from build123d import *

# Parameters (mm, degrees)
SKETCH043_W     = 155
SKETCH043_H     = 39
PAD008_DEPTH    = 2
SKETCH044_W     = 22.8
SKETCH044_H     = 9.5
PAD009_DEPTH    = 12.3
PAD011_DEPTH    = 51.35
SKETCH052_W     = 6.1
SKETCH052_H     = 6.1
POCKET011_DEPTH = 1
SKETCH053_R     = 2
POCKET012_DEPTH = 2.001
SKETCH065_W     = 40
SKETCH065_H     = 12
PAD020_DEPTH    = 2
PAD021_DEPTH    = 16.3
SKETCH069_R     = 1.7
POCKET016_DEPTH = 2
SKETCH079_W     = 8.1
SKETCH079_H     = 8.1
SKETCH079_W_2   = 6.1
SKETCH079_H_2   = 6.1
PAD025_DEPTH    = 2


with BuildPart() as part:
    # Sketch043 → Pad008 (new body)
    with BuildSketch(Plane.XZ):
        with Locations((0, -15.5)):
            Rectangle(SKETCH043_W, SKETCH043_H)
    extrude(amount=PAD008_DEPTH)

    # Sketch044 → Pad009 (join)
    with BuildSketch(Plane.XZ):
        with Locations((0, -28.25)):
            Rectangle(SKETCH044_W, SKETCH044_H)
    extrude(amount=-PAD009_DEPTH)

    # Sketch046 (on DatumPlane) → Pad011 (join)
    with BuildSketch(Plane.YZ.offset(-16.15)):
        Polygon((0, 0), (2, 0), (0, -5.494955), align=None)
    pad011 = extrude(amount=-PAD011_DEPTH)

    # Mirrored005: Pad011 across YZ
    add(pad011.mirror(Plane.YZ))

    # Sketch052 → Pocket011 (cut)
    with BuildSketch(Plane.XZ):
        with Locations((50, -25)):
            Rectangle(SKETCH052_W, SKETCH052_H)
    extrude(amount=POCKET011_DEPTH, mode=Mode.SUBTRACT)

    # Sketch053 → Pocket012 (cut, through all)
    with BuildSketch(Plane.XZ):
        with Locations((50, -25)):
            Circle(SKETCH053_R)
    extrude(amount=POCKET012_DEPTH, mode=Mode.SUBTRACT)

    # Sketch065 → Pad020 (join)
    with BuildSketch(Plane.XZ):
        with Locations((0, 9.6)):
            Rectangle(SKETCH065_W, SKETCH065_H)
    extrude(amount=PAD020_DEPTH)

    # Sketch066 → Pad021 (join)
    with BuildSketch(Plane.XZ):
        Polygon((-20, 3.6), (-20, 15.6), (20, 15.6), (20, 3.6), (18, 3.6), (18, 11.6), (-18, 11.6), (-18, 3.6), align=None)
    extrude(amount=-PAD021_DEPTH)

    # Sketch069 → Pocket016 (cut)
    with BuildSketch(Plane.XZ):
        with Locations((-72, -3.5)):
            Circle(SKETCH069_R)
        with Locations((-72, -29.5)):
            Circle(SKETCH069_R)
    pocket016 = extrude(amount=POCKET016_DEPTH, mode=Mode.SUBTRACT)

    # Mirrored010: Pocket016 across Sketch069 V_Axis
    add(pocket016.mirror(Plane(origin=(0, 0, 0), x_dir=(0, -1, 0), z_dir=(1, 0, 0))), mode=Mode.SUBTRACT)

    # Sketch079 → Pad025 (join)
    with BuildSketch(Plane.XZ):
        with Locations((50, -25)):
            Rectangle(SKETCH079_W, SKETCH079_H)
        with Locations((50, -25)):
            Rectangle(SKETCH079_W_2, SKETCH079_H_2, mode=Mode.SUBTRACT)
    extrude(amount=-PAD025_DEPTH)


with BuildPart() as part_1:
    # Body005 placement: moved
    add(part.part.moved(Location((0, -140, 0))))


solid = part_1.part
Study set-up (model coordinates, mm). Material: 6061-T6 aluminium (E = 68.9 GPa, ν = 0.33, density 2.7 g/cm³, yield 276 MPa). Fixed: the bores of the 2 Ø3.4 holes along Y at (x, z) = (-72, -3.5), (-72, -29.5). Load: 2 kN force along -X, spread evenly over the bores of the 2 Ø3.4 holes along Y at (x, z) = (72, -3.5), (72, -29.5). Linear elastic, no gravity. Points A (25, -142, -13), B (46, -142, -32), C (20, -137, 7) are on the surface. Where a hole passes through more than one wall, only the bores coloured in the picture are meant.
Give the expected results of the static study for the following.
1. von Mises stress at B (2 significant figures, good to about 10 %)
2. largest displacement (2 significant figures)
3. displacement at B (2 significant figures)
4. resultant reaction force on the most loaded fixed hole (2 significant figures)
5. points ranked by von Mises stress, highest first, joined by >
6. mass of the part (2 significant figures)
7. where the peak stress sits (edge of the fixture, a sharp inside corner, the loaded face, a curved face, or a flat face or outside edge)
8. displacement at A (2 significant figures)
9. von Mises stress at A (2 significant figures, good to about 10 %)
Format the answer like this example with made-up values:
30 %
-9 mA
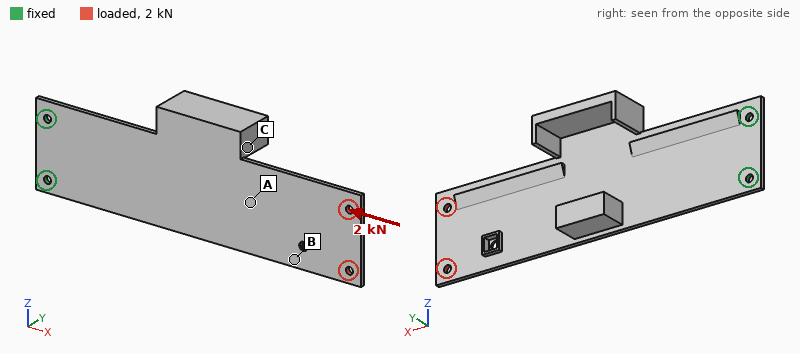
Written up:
39 MPa
0.55 mm
0.34 mm
1.0 kN
B > A > C
52 g
the loaded face
0.23 mm
26 MPa
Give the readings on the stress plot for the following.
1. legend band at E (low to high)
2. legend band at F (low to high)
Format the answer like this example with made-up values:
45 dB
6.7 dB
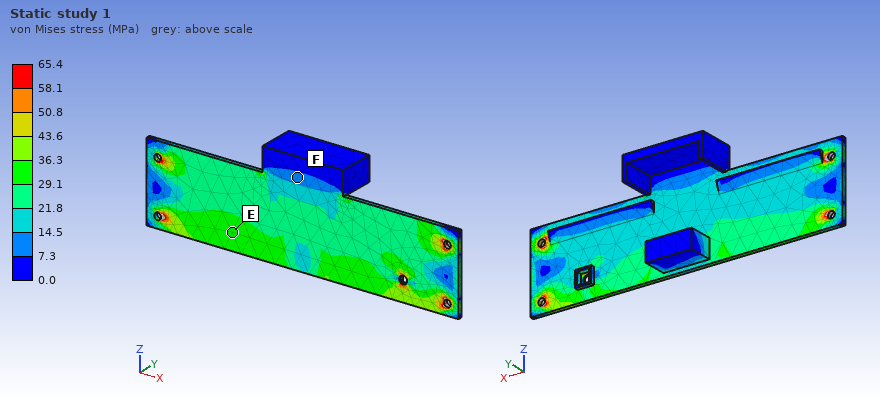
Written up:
29.1 to 36.3 MPa
7.3 to 14.5 MPa
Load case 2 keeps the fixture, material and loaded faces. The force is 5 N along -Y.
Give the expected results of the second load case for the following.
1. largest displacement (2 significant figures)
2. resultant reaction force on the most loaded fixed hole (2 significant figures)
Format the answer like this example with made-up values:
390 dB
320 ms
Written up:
1.9 mm
8.3 N
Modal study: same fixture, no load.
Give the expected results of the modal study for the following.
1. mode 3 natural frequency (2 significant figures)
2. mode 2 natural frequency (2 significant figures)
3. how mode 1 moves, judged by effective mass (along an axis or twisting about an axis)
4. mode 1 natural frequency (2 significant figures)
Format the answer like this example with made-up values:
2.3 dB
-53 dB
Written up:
480 Hz
340 Hz
along Y
77 Hz
